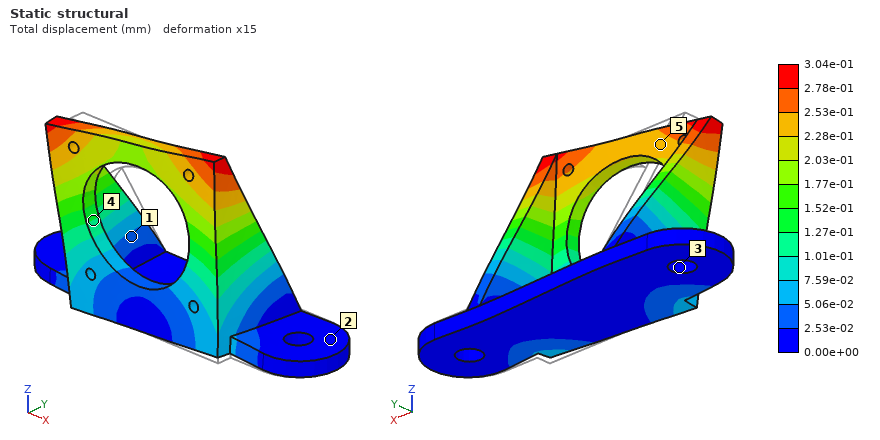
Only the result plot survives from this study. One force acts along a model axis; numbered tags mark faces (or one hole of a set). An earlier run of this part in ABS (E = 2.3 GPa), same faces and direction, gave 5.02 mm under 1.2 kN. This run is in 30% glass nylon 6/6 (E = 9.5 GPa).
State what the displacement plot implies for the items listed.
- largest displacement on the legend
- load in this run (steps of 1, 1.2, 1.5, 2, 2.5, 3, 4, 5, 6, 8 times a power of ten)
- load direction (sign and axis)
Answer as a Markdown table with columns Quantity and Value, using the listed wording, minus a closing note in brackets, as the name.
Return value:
| Quantity | Value |
|---|---|
| largest displacement on the legend | 3.04e-01 mm |
| load in this run | 300 N |
| load direction | -X |
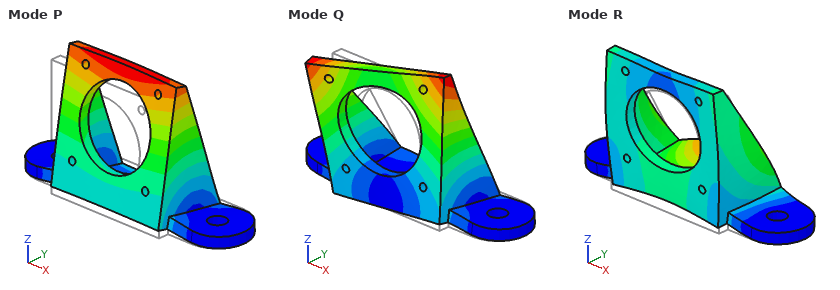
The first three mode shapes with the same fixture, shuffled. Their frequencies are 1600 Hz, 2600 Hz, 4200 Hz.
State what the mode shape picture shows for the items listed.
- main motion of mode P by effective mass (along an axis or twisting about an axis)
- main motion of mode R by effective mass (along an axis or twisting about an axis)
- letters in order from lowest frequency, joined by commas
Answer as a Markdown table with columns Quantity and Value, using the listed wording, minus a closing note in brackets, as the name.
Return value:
| Quantity | Value |
|---|---|
| main motion of mode P by effective mass | along Y |
| main motion of mode R by effective mass | along Z |
| letters in order from lowest frequency, joined by commas | P, Q, R |
